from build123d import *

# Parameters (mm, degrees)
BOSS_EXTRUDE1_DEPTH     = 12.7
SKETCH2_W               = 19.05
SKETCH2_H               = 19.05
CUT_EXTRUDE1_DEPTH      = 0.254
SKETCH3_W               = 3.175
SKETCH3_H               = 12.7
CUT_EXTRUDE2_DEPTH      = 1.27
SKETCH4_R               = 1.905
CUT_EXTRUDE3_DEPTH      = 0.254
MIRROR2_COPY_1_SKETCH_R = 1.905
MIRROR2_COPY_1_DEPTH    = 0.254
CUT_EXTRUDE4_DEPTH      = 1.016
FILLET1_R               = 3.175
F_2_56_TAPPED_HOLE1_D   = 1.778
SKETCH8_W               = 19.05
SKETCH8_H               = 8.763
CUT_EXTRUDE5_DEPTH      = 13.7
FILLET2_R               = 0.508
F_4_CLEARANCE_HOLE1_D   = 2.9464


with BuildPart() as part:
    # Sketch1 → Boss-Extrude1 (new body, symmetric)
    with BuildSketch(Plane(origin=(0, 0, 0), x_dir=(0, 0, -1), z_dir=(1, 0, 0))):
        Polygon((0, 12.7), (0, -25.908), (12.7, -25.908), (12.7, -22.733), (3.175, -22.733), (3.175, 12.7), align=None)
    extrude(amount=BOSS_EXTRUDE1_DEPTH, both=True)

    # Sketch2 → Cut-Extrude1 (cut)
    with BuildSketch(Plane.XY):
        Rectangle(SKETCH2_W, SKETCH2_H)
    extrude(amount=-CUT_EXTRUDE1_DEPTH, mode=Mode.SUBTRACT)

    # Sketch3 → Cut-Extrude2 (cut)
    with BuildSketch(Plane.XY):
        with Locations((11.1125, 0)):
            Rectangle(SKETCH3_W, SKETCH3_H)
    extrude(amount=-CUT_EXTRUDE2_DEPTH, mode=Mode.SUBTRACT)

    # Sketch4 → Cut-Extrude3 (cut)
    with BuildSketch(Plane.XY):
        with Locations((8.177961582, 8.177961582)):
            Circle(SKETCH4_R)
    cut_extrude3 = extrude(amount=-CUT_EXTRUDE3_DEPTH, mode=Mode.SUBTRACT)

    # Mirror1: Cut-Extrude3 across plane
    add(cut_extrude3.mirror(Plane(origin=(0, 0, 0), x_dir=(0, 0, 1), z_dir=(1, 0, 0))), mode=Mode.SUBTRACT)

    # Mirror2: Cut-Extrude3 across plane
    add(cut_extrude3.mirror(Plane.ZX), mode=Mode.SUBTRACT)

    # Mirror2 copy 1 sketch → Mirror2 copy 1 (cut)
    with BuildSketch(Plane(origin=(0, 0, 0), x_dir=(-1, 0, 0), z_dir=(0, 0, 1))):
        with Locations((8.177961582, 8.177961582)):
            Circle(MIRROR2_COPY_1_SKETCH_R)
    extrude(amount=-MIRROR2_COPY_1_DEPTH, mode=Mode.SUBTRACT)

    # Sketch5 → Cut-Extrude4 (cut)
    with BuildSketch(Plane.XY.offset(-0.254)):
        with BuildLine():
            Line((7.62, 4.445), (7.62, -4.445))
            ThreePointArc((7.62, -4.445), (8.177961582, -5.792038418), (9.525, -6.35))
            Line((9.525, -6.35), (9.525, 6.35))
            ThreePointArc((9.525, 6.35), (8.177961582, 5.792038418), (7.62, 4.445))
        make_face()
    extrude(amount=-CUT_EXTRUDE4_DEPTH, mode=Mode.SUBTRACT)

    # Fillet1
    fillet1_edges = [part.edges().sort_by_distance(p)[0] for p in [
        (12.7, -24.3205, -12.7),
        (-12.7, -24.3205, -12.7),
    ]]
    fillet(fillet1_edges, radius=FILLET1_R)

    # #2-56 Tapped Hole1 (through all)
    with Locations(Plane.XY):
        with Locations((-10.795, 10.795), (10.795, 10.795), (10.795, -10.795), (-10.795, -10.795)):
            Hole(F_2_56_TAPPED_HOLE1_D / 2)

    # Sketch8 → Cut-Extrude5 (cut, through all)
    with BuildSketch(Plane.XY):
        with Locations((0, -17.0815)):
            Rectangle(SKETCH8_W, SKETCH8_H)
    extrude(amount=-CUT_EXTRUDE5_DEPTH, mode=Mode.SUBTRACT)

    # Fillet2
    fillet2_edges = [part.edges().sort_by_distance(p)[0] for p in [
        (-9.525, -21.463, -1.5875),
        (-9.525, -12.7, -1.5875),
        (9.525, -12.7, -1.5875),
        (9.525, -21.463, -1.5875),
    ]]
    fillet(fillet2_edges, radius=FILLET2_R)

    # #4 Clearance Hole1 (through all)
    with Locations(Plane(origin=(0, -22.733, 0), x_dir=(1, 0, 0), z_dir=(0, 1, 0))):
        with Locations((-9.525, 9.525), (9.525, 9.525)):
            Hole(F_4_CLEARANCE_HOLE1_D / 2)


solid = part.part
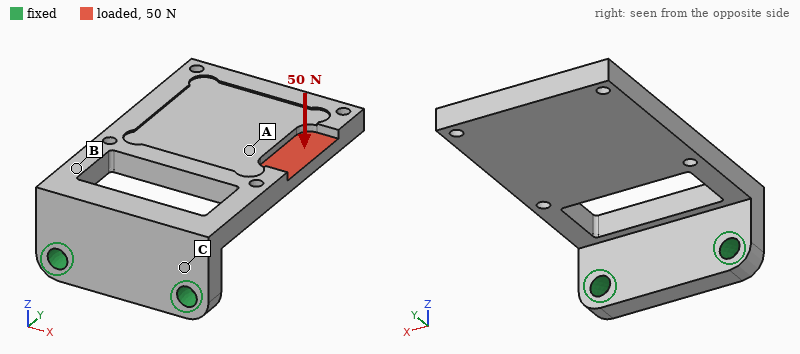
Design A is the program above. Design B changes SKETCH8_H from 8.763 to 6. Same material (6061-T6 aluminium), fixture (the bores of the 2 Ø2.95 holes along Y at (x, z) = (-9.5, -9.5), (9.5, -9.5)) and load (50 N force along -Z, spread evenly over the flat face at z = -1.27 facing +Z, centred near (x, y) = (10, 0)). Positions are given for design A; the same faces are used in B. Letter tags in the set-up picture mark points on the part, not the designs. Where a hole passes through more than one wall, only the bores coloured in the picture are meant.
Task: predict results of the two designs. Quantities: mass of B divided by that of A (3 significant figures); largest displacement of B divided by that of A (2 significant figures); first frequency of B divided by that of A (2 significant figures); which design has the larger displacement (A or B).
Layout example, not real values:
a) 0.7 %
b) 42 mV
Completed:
a) 1.05
b) 0.88
c) 1.1
d) A
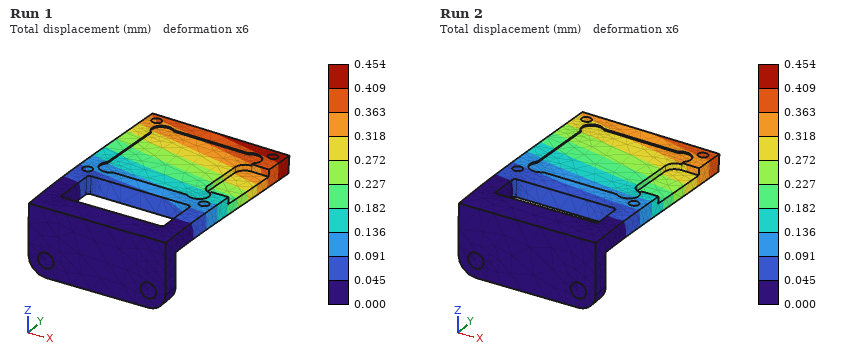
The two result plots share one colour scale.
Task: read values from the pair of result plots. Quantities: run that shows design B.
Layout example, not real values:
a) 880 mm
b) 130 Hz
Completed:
a) Run 2
